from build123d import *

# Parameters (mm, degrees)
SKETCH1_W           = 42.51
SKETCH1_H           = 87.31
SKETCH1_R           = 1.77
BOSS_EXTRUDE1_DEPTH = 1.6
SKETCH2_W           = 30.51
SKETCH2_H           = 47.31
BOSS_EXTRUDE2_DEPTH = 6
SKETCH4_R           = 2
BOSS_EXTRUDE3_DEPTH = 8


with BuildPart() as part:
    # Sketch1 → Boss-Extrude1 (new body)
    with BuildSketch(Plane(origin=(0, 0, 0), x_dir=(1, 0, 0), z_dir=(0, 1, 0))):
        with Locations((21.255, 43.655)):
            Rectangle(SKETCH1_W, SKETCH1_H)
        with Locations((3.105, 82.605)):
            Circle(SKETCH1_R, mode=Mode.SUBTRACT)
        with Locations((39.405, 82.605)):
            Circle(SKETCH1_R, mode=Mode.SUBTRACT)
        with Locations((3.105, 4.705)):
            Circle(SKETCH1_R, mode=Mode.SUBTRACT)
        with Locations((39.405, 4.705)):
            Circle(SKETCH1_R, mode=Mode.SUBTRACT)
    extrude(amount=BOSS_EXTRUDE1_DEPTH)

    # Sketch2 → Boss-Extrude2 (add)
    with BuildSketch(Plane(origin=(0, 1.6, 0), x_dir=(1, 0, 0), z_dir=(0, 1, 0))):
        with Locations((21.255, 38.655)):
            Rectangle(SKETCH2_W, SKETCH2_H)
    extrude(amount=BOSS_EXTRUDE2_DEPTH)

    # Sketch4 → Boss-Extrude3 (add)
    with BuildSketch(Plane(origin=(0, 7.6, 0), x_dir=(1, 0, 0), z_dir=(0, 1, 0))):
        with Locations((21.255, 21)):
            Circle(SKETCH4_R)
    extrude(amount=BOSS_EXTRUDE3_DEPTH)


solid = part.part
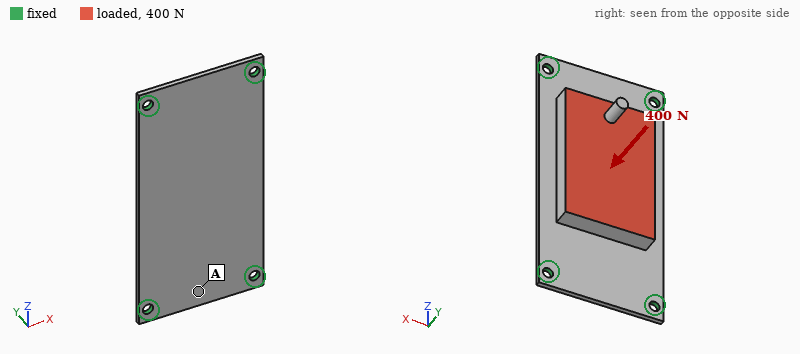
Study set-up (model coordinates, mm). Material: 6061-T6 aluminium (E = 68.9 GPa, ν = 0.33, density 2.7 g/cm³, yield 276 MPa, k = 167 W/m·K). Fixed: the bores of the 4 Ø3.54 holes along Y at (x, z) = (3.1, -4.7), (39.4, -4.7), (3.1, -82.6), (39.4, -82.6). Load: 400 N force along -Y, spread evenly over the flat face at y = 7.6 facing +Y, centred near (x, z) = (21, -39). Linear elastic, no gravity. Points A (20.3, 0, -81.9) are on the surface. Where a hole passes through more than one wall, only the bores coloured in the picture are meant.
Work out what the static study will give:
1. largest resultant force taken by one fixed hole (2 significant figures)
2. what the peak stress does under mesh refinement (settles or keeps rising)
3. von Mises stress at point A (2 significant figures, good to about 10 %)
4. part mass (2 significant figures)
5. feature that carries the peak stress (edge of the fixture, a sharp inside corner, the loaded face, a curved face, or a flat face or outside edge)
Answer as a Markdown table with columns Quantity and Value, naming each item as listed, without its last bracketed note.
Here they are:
| Quantity | Value |
|---|---|
| largest resultant force taken by one fixed hole | 170 N |
| what the peak stress does under mesh refinement | keeps rising |
| von Mises stress at point A | 20 MPa |
| part mass | 40 g |
| feature that carries the peak stress | edge of the fixture |
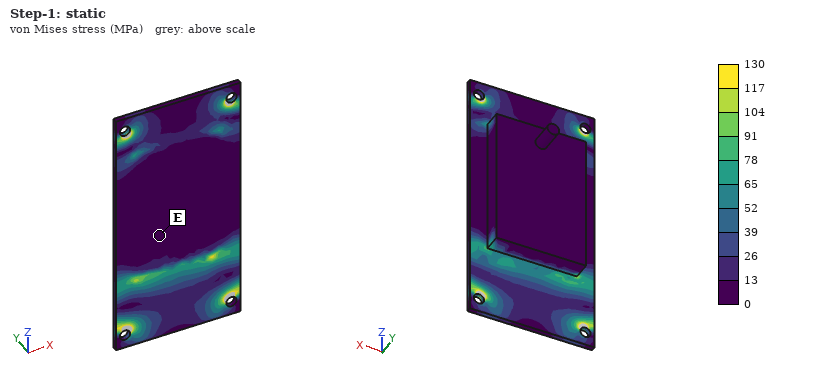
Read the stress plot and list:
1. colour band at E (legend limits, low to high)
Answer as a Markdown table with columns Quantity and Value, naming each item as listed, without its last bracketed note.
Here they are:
| Quantity | Value |
|---|---|
| colour band at E | 0 to 13 MPa |
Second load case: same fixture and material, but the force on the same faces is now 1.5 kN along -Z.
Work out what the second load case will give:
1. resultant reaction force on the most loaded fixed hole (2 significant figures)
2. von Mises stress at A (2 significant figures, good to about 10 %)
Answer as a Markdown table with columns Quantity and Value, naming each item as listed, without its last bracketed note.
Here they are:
| Quantity | Value |
|---|---|
| resultant reaction force on the most loaded fixed hole | 430 N |
| von Mises stress at A | 19 MPa |
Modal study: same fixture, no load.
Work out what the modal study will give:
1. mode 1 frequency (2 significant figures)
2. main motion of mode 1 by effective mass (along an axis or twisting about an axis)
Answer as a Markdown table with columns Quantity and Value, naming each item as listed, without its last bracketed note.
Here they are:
| Quantity | Value |
|---|---|
| mode 1 frequency | 1500 Hz |
| main motion of mode 1 by effective mass | along Y |
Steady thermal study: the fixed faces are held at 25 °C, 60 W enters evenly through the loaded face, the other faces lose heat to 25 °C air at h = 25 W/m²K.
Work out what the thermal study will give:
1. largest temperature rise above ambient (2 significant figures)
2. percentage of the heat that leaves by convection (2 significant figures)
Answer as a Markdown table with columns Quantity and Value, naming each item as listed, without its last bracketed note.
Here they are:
| Quantity | Value |
|---|---|
| largest temperature rise above ambient | 61 K |
| percentage of the heat that leaves by convection | 13 % |
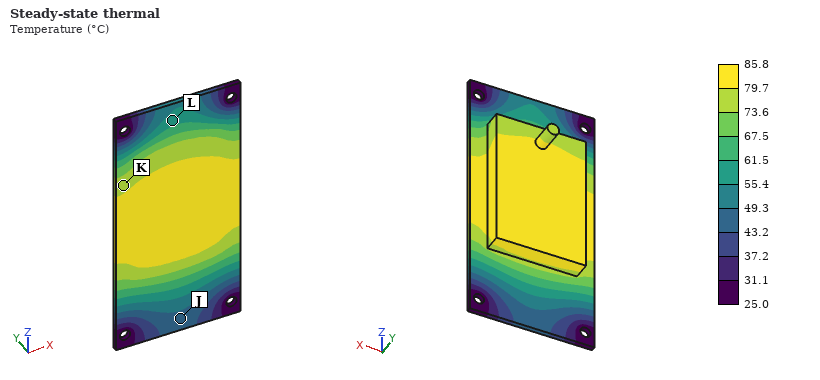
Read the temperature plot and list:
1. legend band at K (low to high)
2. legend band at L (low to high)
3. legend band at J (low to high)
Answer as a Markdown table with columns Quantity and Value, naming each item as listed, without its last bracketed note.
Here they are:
| Quantity | Value |
|---|---|
| legend band at K | 73.6 to 79.7 °C |
| legend band at L | 55.4 to 61.5 °C |
| legend band at J | 43.2 to 49.3 °C |
